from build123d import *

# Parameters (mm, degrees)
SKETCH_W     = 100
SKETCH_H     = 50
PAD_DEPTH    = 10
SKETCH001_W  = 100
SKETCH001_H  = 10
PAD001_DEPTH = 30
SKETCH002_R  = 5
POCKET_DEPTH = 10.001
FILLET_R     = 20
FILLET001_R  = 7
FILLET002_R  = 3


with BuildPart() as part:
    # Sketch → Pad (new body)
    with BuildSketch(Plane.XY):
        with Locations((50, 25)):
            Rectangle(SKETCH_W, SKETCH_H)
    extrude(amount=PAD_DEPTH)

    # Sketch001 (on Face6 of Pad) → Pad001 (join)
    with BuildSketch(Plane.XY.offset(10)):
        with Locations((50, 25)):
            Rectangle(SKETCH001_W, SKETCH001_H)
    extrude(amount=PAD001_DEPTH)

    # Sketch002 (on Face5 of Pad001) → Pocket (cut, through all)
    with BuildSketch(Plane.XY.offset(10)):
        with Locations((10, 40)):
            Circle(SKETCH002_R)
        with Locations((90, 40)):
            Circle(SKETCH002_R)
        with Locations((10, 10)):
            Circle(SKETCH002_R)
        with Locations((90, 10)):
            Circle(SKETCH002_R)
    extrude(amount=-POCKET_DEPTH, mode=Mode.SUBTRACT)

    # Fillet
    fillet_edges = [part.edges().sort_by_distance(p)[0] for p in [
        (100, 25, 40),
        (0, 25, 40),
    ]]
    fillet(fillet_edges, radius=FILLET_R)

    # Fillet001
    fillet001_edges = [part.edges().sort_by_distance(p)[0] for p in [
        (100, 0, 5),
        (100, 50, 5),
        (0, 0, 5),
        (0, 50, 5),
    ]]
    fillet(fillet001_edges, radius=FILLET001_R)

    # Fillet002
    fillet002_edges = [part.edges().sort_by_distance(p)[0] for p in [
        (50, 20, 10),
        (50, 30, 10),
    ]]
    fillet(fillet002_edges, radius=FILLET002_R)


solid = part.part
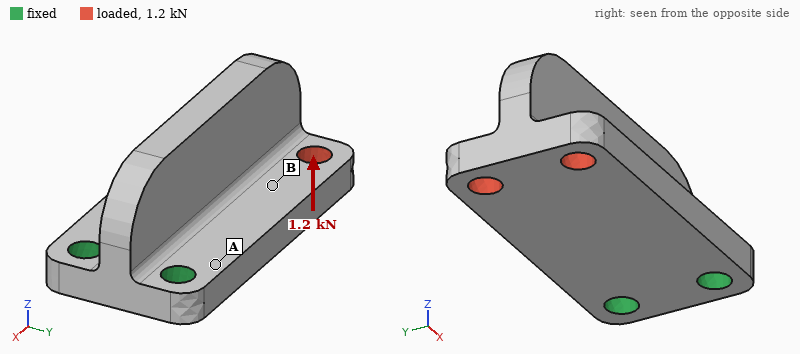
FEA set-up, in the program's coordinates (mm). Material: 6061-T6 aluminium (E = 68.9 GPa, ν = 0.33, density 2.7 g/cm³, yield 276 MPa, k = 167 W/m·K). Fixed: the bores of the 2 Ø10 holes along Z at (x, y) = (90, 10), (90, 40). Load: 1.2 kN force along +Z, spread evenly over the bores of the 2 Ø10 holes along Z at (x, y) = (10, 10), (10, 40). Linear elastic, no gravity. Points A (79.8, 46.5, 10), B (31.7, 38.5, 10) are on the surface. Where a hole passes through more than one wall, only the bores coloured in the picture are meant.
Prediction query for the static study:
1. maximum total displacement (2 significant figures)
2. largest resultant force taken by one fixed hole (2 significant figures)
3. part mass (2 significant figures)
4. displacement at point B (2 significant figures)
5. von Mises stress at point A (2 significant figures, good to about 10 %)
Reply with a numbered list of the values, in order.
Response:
1. 0.21 mm
2. 600 N
3. 200 g
4. 0.12 mm
5. 40 MPa
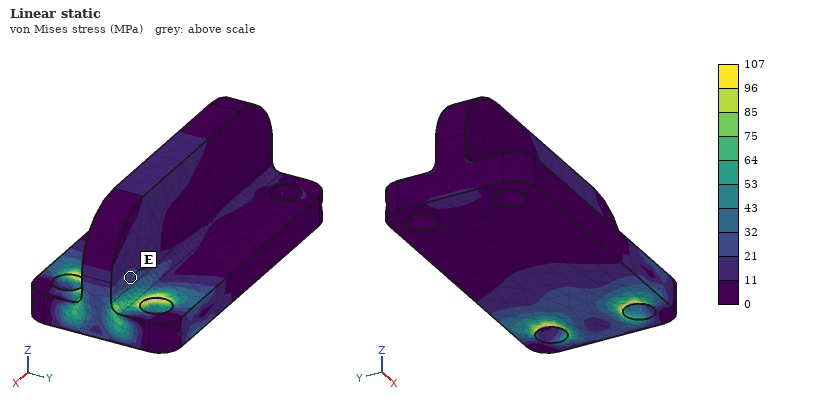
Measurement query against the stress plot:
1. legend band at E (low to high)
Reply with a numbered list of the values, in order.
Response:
1. 21 to 32 MPa
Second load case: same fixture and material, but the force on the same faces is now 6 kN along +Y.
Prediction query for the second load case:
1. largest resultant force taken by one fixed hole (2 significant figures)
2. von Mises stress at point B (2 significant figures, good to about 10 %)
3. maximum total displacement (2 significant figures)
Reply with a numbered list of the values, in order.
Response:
1. 14 kN
2. 24 MPa
3. 0.21 mm
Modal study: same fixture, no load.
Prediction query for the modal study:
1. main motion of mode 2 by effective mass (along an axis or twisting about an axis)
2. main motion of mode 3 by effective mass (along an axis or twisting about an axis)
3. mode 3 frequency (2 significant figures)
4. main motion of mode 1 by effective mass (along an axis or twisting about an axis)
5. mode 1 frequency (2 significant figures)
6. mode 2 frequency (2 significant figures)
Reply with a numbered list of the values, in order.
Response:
1. along Y
2. along Y
3. 4300 Hz
4. along Z
5. 1500 Hz
6. 3000 Hz
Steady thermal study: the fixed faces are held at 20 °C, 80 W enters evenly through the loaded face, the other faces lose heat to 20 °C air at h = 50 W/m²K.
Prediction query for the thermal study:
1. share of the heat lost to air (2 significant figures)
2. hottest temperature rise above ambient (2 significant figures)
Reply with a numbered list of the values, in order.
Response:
1. 24 %
2. 52 K
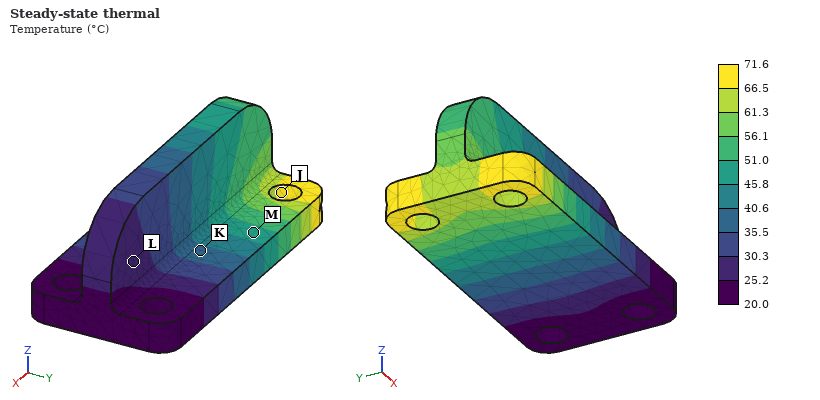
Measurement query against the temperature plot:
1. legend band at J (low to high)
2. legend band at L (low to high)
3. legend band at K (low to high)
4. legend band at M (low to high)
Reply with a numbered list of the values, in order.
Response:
1. 66.5 to 71.6 °C
2. 25.2 to 30.3 °C
3. 35.5 to 40.6 °C
4. 45.8 to 51.0 °C
